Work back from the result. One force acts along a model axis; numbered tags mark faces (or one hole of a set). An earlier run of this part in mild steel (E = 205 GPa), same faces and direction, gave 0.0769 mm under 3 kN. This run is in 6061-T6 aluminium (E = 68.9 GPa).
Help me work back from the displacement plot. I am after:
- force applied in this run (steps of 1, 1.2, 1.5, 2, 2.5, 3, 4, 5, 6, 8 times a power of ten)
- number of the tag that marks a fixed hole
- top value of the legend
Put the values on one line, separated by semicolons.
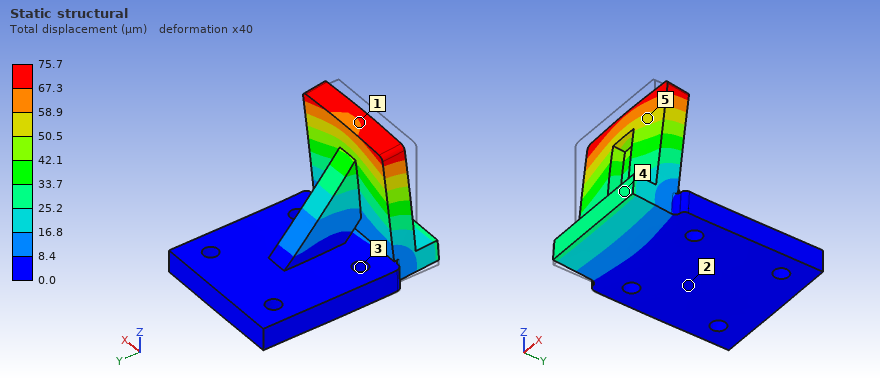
1 kN; 3; 75.7 µm
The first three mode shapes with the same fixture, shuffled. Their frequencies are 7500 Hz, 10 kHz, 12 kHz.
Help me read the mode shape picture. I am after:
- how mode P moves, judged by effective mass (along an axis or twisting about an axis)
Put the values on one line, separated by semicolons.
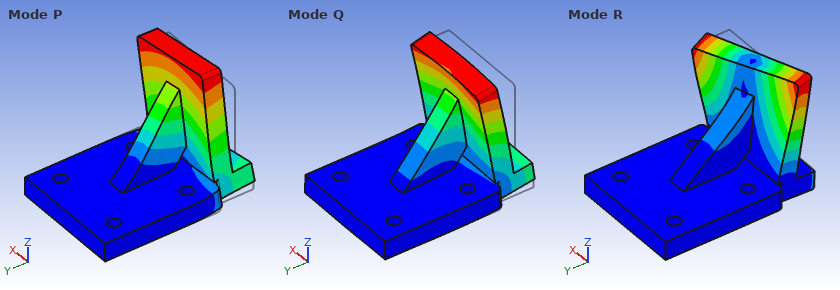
along X
